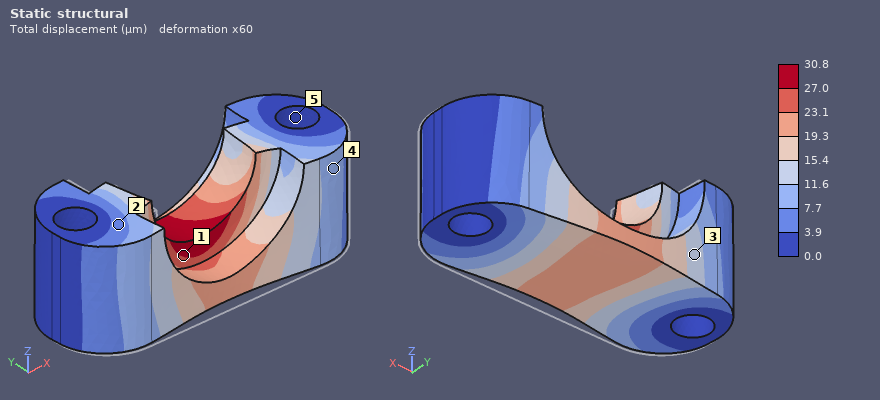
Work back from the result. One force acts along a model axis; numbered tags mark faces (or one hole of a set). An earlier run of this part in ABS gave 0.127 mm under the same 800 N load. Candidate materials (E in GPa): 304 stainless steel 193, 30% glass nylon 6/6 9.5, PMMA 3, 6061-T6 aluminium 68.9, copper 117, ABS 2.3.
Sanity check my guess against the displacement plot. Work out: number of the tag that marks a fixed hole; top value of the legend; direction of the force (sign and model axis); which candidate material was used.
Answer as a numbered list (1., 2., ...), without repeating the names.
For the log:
1. 5
2. 30.8 µm
3. +Y
4. 30% glass nylon 6/6
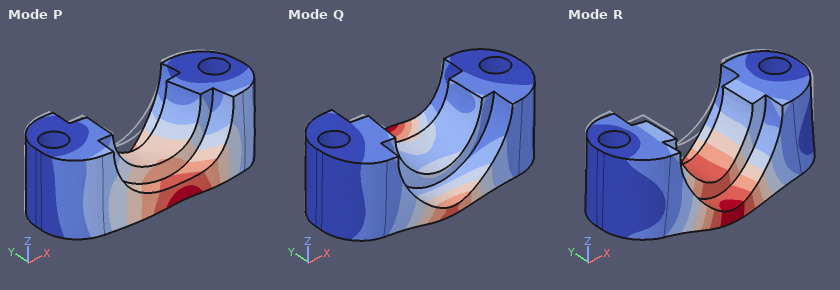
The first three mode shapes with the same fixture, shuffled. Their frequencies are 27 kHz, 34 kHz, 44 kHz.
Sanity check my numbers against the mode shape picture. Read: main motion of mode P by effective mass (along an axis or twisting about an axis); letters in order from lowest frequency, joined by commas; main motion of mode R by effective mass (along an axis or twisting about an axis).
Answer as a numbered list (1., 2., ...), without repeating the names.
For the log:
1. along Y
2. P, R, Q
3. along Z
